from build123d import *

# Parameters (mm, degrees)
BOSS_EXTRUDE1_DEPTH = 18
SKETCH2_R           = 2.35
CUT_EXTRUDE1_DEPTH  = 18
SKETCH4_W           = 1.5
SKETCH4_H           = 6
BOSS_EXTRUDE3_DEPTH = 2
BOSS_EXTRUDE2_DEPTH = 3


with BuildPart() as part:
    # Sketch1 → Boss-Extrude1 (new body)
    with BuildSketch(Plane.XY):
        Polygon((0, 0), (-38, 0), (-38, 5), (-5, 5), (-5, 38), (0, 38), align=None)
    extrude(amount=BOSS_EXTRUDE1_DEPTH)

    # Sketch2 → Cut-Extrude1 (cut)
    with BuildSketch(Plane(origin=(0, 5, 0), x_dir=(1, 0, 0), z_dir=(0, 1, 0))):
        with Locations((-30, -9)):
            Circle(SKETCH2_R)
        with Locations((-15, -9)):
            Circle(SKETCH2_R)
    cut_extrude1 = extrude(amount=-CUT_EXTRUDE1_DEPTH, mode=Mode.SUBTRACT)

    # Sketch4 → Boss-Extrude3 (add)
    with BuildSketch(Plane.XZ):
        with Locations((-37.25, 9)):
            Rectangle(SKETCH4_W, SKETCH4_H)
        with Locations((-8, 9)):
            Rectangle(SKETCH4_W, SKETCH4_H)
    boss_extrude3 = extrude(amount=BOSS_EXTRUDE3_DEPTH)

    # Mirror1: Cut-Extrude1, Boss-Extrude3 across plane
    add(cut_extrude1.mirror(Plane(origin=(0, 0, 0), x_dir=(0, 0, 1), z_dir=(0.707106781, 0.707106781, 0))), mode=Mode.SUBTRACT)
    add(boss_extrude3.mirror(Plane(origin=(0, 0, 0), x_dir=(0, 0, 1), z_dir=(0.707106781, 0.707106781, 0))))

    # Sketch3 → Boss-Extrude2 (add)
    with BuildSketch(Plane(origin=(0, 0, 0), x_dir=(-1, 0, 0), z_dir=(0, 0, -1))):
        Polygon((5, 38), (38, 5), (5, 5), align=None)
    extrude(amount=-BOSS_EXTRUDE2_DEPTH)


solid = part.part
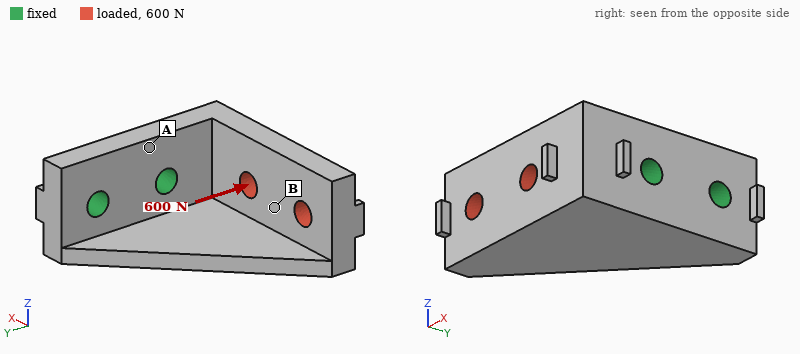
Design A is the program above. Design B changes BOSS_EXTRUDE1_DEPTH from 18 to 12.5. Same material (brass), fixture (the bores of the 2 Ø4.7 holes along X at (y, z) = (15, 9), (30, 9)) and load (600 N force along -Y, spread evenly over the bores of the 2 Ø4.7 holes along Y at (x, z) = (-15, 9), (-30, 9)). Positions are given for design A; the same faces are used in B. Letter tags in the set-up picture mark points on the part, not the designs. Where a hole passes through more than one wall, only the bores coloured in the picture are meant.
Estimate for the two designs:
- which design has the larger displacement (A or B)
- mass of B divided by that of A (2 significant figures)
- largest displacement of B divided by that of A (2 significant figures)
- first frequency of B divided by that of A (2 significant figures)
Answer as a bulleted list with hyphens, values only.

- B
- 0.75
- 1.3
- 0.92
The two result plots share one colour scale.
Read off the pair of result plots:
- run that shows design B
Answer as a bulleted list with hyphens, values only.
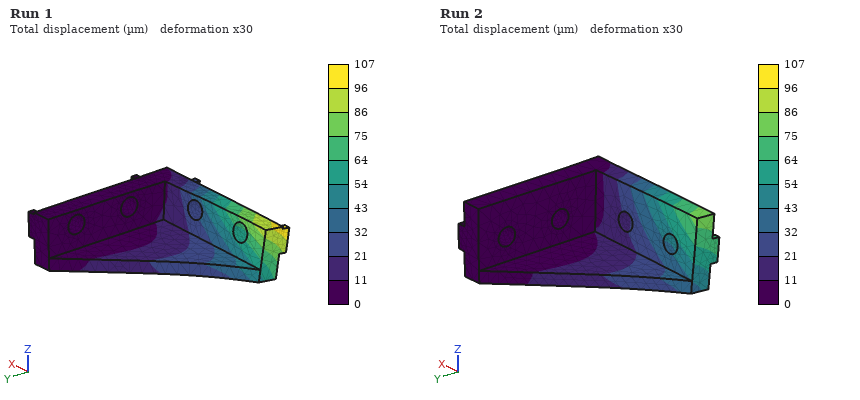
- Run 1
